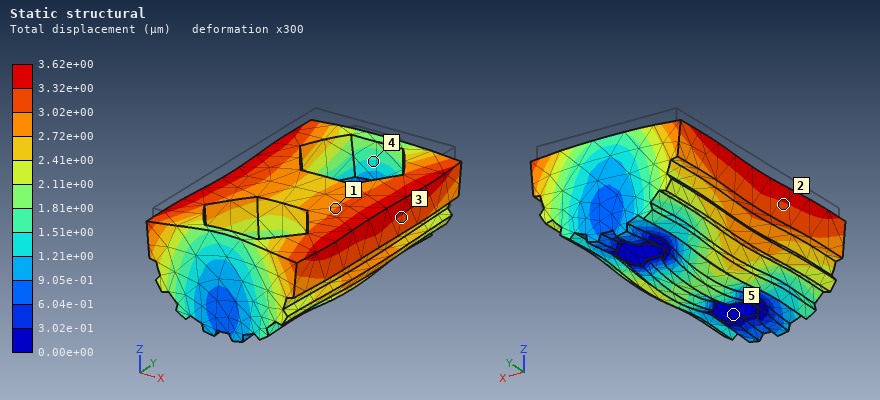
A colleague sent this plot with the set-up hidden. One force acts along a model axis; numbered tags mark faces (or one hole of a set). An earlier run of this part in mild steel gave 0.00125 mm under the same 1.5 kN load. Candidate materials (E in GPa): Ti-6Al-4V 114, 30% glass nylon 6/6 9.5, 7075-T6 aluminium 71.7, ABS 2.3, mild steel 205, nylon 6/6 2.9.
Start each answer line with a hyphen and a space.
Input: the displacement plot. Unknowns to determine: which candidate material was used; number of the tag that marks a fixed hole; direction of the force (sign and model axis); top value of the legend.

- 7075-T6 aluminium
- 5
- -Z
- 3.62e+00 µm
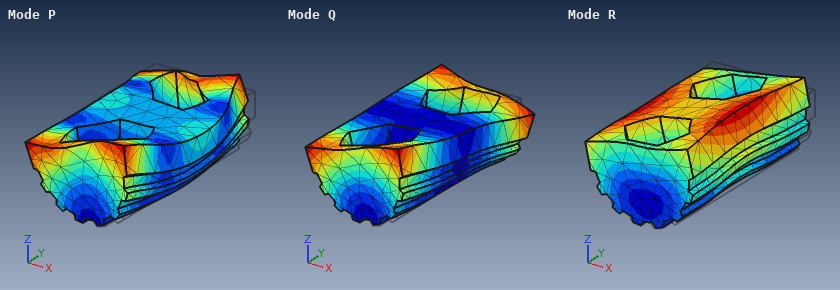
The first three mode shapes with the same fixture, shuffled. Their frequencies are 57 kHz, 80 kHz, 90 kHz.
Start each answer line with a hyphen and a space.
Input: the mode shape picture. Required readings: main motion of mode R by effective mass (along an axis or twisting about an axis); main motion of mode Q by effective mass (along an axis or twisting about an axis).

- along X
- twisting about Z
